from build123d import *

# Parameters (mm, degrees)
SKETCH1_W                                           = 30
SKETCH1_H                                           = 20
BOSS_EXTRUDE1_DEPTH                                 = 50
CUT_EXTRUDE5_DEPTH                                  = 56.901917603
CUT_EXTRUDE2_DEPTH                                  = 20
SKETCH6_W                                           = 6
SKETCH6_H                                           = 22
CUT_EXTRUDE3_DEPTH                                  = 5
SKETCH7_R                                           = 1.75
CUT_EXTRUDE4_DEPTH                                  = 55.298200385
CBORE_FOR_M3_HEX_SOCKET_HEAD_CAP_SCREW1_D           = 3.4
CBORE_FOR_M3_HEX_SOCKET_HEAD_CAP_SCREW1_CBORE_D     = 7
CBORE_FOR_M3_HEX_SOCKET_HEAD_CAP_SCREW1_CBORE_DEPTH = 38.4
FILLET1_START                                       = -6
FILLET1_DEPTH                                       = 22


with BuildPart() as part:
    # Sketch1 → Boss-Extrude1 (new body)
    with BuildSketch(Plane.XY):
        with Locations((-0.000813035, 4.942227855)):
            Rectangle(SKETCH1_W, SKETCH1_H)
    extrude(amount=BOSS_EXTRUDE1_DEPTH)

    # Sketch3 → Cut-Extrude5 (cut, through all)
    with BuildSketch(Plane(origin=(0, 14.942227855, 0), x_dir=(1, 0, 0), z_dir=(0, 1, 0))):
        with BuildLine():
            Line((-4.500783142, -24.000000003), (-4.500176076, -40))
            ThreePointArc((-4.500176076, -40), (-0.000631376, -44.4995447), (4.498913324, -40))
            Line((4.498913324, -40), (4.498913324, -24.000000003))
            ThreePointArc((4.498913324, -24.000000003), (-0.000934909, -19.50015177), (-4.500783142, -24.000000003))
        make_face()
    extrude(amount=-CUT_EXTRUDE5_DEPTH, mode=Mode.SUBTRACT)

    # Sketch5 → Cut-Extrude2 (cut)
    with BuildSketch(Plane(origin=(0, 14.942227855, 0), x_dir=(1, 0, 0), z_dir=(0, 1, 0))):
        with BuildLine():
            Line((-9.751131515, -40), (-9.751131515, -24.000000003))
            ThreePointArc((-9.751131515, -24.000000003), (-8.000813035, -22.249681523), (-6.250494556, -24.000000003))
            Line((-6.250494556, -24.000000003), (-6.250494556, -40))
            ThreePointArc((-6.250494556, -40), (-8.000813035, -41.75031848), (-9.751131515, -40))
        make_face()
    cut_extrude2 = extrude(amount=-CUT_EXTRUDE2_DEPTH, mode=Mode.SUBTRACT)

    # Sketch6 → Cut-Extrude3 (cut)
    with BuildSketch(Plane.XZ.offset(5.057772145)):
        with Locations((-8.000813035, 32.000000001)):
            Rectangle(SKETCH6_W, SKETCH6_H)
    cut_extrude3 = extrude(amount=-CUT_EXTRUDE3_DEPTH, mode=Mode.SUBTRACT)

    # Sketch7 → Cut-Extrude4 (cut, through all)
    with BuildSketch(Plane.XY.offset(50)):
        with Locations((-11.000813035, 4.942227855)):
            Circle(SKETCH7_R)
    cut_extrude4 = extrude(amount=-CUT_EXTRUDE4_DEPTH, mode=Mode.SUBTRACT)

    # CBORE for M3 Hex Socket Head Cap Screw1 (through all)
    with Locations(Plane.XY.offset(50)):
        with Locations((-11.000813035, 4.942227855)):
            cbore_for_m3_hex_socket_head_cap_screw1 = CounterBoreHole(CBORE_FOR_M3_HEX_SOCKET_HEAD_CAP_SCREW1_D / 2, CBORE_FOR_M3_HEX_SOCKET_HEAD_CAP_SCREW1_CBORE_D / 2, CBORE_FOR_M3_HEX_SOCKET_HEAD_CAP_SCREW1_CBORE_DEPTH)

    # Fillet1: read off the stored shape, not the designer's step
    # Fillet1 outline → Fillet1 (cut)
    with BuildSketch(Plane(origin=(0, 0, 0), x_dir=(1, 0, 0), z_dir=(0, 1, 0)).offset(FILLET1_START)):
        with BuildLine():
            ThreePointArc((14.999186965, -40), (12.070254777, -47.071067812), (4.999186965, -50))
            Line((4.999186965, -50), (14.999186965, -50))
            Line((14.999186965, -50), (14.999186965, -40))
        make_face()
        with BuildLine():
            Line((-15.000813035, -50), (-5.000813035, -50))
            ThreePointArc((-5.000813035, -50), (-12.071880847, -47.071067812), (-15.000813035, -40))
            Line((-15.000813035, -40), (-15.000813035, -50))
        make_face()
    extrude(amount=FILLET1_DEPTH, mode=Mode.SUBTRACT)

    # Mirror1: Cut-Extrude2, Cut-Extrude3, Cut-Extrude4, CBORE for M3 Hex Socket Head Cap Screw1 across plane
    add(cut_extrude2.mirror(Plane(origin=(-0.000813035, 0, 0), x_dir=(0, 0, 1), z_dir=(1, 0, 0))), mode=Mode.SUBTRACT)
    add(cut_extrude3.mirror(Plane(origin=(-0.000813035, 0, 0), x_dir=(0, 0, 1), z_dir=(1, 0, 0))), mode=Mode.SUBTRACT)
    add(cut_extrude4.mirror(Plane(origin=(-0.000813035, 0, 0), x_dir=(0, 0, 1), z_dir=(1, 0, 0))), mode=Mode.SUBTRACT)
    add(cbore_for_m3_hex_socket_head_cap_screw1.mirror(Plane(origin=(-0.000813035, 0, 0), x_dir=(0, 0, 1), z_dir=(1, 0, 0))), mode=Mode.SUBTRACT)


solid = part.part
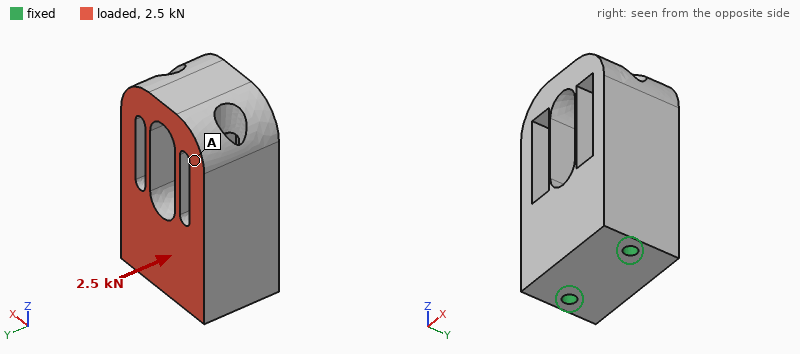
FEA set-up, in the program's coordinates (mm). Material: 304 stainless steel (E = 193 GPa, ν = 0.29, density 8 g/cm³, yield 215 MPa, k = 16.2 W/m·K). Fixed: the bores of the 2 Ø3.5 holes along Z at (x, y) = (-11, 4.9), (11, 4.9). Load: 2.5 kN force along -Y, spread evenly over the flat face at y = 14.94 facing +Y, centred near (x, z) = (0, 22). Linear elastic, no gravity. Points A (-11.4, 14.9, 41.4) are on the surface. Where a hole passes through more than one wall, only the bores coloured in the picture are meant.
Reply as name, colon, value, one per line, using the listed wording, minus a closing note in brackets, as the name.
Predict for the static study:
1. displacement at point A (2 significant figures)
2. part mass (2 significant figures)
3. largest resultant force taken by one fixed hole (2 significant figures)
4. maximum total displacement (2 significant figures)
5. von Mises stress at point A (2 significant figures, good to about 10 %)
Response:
displacement at point A: 17 µm
part mass: 150 g
largest resultant force taken by one fixed hole: 1.3 kN
maximum total displacement: 22 µm
von Mises stress at point A: 8.2 MPa
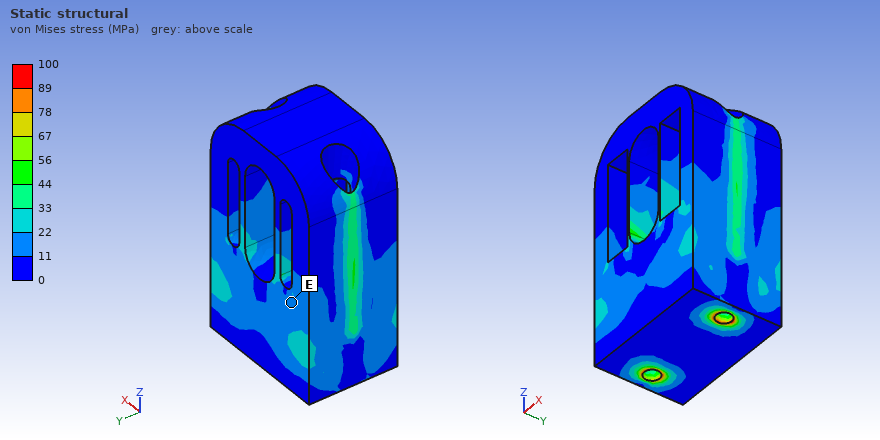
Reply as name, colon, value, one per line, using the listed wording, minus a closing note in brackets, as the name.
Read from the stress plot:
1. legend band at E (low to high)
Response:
legend band at E: 11 to 22 MPa
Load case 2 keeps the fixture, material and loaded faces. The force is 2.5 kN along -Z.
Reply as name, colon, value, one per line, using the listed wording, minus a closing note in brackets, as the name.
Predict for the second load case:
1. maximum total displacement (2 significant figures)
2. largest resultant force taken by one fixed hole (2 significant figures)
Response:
maximum total displacement: 13 µm
largest resultant force taken by one fixed hole: 1.3 kN
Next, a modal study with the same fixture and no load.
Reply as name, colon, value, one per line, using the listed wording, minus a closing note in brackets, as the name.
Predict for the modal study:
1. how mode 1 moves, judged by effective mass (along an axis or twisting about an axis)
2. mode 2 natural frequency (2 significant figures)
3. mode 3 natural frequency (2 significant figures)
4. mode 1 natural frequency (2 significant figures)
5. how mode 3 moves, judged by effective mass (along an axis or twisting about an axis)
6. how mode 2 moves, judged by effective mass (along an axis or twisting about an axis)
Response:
how mode 1 moves, judged by effective mass: along X
mode 2 natural frequency: 5400 Hz
mode 3 natural frequency: 10 kHz
mode 1 natural frequency: 4900 Hz
how mode 3 moves, judged by effective mass: twisting about Z
how mode 2 moves, judged by effective mass: along Y
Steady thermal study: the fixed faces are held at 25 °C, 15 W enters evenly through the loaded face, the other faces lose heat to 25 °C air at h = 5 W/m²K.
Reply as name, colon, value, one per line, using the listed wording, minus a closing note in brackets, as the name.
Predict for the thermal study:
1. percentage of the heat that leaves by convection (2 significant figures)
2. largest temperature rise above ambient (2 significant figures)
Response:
percentage of the heat that leaves by convection: 7.8 %
largest temperature rise above ambient: 55 K
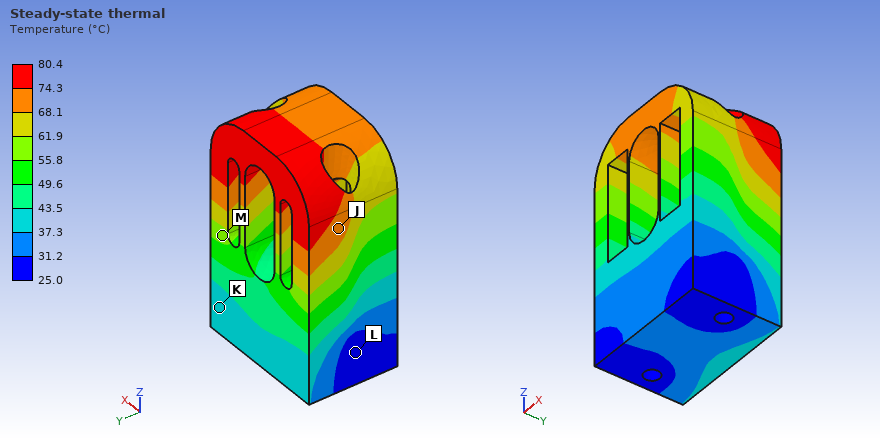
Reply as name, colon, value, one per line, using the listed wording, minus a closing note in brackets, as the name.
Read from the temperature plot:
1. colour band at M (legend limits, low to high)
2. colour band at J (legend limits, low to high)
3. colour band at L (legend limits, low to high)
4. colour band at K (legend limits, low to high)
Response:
colour band at M: 55.8 to 61.9 °C
colour band at J: 68.1 to 74.3 °C
colour band at L: 25.0 to 31.2 °C
colour band at K: 37.3 to 43.5 °C
